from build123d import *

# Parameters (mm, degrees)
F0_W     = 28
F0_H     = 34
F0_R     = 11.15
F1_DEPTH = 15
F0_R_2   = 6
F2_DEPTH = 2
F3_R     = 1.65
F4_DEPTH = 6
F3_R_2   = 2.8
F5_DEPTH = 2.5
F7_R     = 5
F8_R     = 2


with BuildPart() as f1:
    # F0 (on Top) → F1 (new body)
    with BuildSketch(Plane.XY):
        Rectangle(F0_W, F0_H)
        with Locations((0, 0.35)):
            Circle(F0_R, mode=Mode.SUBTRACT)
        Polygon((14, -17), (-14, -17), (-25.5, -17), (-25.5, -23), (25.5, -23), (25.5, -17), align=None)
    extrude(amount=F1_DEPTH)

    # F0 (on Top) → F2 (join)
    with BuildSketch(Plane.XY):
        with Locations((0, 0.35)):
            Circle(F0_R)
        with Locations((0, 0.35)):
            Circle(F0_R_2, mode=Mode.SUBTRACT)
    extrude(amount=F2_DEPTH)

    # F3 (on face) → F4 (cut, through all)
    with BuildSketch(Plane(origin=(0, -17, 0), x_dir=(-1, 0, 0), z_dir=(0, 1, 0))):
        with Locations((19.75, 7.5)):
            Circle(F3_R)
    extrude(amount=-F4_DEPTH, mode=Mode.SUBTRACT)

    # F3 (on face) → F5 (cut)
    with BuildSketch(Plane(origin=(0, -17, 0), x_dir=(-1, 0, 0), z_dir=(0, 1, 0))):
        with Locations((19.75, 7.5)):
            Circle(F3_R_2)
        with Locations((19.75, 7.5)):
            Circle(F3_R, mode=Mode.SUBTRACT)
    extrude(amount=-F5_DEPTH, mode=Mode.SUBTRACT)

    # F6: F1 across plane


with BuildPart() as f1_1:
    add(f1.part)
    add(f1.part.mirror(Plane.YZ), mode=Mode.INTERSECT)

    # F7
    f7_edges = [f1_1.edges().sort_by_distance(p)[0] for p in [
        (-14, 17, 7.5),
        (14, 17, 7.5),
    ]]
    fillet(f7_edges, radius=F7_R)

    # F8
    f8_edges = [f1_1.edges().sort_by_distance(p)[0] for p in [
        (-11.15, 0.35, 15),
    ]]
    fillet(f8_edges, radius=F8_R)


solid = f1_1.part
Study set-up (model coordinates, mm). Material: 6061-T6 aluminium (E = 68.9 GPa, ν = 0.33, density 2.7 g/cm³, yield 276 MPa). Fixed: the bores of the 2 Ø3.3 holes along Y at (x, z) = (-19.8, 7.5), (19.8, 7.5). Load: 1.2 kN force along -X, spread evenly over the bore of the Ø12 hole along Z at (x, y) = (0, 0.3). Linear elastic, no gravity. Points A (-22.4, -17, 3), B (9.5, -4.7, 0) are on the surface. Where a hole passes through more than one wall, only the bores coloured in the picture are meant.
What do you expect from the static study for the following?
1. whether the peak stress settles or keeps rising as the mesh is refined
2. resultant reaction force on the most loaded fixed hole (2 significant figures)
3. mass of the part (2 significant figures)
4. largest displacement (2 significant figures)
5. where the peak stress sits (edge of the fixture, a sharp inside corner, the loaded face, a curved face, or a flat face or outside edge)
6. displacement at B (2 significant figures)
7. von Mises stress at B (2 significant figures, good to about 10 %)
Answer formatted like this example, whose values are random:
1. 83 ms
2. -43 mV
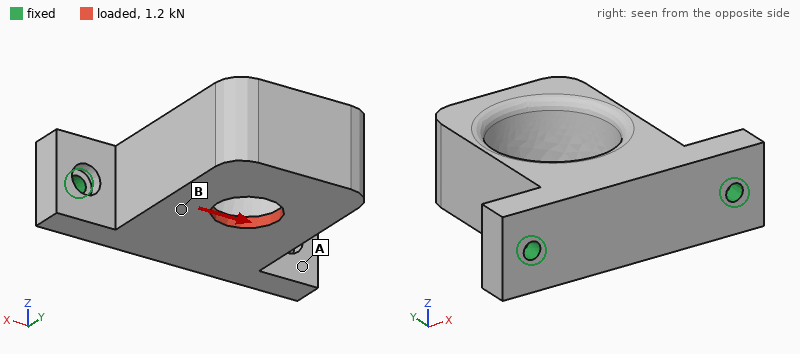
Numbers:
1. keeps rising
2. 950 N
3. 36 g
4. 35 µm
5. edge of the fixture
6. 15 µm
7. 31 MPa
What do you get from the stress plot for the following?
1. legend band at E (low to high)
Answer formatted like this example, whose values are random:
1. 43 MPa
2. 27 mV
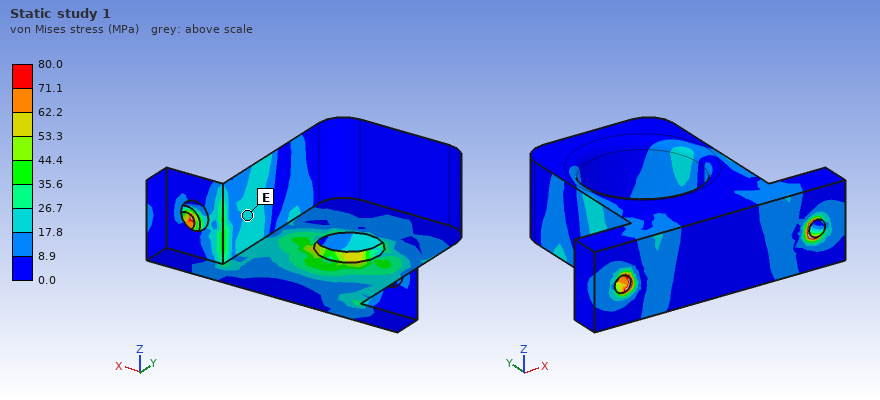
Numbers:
1. 17.8 to 26.7 MPa
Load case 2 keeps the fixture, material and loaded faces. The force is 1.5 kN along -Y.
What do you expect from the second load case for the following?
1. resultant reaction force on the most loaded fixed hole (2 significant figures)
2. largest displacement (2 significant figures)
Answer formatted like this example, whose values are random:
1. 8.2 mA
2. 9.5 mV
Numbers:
1. 910 N
2. 0.13 mm
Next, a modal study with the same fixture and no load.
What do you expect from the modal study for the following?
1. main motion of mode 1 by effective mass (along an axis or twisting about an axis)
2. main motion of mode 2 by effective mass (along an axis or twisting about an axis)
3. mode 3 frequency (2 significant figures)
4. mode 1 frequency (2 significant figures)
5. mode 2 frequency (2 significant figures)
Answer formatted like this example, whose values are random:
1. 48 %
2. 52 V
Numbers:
1. along Z
2. along X
3. 12 kHz
4. 2300 Hz
5. 6400 Hz
